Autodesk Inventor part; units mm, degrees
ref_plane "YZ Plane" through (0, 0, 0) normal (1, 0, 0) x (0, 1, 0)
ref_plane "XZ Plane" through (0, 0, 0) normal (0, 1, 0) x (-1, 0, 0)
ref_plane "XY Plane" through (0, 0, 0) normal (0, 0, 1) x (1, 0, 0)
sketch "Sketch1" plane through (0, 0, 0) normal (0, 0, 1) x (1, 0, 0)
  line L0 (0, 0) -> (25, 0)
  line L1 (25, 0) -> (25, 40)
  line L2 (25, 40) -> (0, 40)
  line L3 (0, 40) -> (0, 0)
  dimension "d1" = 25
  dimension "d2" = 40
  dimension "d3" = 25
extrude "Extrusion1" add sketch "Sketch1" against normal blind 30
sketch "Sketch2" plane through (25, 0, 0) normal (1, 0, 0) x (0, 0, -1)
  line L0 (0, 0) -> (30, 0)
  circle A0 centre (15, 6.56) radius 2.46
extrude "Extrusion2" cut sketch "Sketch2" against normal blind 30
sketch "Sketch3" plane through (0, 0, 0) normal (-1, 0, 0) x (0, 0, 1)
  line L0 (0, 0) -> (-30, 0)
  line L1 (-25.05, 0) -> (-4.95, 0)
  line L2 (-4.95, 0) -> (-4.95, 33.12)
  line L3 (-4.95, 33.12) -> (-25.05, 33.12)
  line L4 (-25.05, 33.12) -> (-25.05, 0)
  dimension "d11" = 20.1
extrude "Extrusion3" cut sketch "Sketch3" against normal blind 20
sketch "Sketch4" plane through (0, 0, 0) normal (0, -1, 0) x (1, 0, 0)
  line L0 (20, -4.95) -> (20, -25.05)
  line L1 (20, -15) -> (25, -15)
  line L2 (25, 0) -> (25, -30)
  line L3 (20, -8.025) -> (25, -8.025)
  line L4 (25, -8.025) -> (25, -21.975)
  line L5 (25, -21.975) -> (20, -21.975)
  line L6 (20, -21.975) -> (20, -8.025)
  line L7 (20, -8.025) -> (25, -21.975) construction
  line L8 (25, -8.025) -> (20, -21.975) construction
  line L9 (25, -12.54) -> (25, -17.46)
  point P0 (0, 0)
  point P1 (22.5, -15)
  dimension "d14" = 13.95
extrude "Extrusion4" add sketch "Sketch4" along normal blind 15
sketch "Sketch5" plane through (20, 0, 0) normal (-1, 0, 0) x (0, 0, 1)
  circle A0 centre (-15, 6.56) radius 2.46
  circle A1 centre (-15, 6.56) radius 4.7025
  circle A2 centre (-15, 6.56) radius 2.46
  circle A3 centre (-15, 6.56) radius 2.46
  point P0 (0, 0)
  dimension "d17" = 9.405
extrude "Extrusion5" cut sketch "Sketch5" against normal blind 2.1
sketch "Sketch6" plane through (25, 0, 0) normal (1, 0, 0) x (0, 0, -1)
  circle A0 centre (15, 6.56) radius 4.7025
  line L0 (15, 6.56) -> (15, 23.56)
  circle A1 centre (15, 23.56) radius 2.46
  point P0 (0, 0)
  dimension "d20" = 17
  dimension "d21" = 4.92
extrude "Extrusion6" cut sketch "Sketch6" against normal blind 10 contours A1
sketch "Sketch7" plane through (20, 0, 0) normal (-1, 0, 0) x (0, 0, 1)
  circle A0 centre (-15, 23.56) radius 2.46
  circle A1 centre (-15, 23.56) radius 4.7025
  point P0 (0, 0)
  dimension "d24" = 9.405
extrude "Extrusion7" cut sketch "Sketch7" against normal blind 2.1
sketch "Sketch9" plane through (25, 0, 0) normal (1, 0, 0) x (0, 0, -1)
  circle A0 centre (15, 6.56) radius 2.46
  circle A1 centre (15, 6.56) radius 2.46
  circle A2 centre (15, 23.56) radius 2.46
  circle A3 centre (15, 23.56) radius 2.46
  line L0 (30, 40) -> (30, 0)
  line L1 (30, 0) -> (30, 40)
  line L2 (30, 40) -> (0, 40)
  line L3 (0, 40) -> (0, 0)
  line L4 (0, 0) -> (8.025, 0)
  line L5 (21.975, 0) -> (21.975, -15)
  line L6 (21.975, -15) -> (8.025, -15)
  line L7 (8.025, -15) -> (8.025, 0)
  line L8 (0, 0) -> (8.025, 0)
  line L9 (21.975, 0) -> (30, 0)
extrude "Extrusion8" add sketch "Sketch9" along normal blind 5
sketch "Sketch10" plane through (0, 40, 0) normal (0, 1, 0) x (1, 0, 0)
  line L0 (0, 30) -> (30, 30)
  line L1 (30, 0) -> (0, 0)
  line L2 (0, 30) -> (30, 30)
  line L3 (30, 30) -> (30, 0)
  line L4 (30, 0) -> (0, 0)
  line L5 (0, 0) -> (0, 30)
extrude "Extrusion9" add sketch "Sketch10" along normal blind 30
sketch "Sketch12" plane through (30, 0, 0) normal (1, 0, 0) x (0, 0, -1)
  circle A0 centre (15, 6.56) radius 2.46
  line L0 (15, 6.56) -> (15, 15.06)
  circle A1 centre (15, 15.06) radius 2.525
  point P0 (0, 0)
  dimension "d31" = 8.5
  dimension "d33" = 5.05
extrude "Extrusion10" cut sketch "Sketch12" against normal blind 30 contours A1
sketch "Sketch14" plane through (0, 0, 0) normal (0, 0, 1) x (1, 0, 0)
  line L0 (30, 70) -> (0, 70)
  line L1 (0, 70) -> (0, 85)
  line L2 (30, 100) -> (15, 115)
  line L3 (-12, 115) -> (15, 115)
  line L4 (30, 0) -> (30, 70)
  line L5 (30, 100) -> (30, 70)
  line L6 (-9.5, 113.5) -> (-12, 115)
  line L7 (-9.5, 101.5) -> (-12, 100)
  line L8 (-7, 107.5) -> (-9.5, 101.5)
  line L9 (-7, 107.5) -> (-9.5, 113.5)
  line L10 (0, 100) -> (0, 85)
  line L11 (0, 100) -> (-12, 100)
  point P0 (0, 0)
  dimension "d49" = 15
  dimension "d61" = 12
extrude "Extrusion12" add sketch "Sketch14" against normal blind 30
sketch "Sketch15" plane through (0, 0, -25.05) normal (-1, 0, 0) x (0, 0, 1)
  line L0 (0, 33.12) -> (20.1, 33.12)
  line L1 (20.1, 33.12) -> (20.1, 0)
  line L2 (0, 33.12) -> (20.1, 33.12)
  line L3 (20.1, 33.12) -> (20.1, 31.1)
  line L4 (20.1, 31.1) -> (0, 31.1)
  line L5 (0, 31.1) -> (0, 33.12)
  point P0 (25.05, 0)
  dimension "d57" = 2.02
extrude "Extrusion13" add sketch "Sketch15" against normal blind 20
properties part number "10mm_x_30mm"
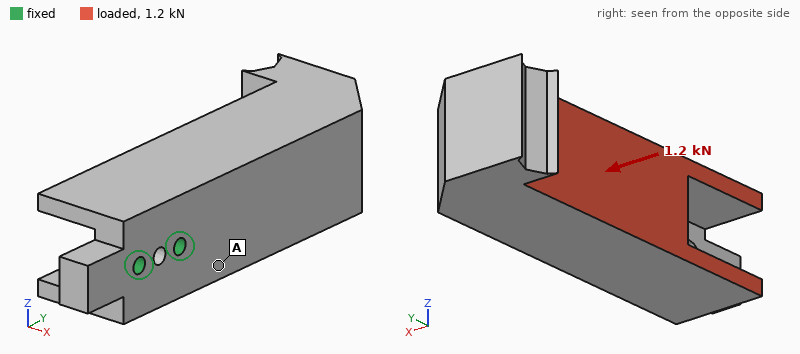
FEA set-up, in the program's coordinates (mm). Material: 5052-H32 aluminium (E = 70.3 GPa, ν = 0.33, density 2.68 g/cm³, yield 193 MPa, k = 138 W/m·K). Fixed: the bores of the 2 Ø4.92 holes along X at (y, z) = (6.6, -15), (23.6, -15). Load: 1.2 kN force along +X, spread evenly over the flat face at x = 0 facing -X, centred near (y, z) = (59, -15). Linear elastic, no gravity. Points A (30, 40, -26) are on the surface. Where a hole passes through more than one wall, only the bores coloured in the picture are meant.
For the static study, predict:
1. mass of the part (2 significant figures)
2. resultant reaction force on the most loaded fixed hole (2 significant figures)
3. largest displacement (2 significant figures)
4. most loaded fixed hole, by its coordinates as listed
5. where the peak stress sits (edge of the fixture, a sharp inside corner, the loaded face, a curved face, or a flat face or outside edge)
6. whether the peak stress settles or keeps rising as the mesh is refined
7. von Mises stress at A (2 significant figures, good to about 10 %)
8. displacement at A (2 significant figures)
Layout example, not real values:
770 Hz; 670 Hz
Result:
250 g; 2.8 kN; 0.11 mm; (23.6, -15); edge of the fixture; keeps rising; 6.7 MPa; 0.020 mm
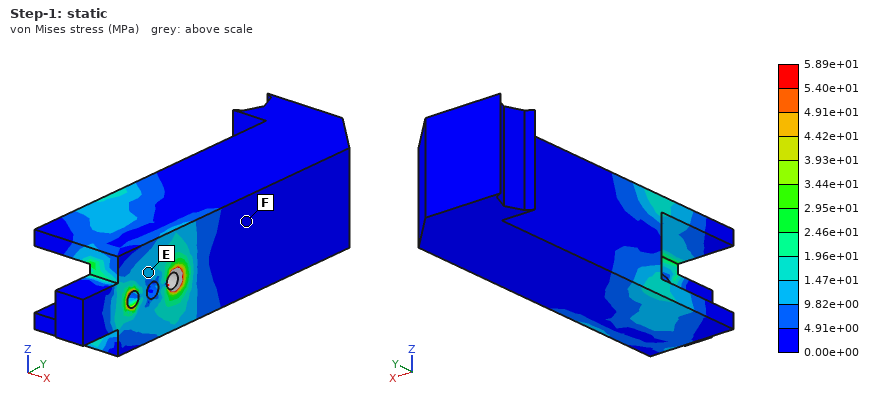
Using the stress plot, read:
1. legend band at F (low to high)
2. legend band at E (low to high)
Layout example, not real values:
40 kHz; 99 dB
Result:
0.00e+00 to 4.91e+00 MPa; 9.82e+00 to 1.47e+01 MPa
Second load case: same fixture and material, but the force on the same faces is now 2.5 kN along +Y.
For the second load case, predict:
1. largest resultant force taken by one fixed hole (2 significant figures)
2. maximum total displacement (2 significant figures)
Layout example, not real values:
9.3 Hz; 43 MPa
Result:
2.9 kN; 0.15 mm
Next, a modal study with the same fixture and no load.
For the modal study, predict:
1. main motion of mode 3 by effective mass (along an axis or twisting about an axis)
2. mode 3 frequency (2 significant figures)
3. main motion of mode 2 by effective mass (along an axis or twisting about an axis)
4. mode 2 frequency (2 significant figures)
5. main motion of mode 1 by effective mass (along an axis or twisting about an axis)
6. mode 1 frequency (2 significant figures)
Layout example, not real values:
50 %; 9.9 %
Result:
twisting about Y; 3500 Hz; along Z; 1400 Hz; along X; 1200 Hz
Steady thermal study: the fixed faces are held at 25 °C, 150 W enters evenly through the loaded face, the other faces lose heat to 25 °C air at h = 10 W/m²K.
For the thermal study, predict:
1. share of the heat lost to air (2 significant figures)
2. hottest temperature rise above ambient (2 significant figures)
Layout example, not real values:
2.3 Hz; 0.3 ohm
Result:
5.0 %; 77 K
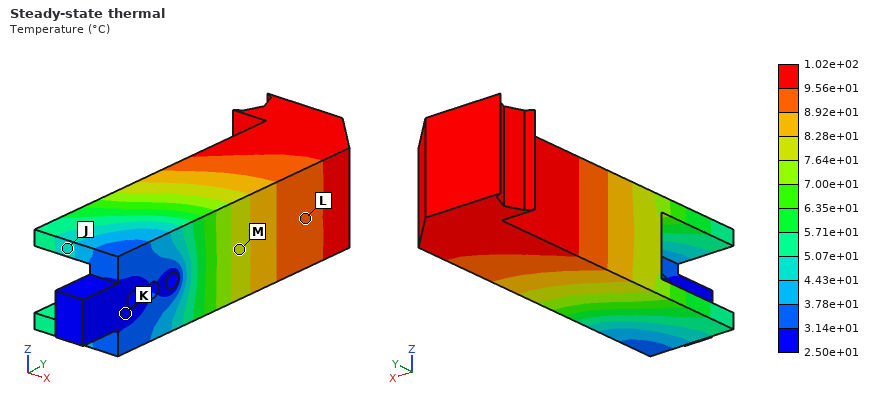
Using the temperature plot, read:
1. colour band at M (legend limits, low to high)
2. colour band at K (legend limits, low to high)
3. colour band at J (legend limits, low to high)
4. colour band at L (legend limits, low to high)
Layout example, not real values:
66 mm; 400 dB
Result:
7.64e+01 to 8.28e+01 °C; 2.50e+01 to 3.14e+01 °C; 4.43e+01 to 5.07e+01 °C; 8.92e+01 to 9.56e+01 °C
